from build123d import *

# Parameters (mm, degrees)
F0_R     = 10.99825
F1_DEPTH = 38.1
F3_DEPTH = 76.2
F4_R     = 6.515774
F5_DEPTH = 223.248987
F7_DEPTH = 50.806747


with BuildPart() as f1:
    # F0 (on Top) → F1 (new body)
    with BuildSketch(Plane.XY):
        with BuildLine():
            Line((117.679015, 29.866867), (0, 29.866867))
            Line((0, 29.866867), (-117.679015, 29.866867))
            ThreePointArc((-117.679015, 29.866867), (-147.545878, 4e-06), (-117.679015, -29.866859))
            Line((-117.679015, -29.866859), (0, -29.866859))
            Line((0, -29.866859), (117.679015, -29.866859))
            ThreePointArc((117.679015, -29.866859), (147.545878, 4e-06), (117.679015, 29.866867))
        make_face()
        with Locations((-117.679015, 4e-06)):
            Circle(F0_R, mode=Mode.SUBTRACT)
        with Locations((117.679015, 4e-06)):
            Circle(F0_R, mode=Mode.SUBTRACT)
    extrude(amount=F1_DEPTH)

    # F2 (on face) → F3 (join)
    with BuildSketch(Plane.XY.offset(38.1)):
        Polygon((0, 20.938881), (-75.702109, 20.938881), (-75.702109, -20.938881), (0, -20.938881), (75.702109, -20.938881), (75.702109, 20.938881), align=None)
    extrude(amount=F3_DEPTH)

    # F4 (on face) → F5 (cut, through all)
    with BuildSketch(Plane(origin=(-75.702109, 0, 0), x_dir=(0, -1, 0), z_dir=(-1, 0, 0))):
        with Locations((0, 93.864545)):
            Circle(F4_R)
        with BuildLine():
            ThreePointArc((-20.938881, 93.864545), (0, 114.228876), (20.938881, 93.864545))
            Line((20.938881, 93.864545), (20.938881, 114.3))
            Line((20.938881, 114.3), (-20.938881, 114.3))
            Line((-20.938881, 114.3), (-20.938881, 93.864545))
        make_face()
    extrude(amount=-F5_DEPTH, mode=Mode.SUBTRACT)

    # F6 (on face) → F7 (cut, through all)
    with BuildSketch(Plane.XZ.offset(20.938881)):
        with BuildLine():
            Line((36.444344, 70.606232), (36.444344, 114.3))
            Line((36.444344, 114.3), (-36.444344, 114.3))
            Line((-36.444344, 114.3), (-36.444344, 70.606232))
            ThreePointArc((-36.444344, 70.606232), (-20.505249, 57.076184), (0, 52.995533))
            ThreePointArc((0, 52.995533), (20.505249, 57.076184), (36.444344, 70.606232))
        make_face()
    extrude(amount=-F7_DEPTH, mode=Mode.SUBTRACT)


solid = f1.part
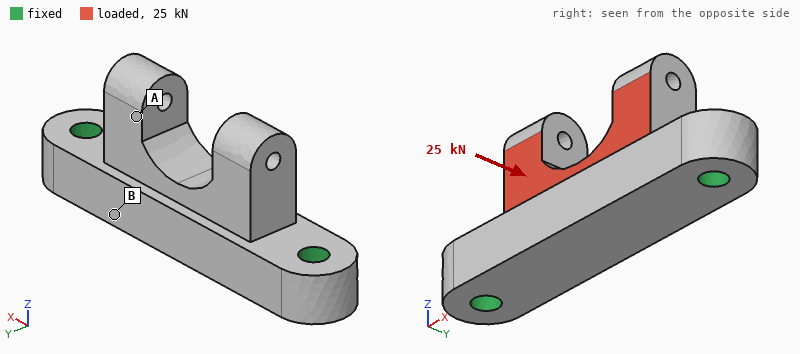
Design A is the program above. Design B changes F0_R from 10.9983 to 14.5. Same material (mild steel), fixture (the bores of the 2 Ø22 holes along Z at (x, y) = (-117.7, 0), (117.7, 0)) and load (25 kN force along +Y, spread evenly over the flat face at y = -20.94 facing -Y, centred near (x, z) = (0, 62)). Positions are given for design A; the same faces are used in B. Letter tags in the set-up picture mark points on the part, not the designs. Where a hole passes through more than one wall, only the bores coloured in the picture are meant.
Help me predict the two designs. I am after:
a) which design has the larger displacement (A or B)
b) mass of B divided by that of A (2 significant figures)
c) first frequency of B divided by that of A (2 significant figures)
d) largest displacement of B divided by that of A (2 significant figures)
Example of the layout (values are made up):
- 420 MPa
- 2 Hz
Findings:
- A
- 0.98
- 1.1
- 0.88
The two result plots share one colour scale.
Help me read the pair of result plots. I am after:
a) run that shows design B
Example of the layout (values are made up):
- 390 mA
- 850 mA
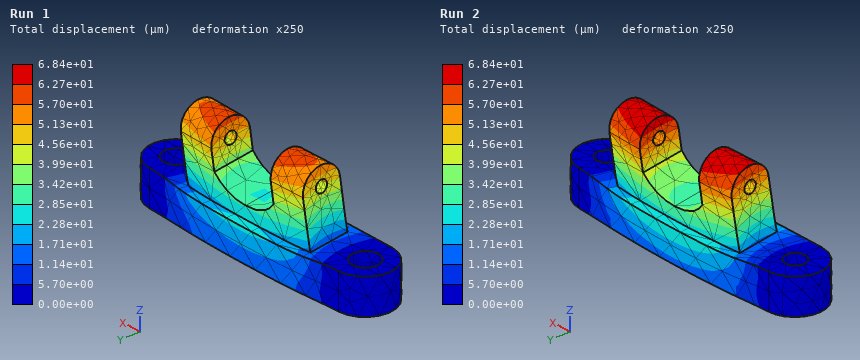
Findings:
- Run 1
